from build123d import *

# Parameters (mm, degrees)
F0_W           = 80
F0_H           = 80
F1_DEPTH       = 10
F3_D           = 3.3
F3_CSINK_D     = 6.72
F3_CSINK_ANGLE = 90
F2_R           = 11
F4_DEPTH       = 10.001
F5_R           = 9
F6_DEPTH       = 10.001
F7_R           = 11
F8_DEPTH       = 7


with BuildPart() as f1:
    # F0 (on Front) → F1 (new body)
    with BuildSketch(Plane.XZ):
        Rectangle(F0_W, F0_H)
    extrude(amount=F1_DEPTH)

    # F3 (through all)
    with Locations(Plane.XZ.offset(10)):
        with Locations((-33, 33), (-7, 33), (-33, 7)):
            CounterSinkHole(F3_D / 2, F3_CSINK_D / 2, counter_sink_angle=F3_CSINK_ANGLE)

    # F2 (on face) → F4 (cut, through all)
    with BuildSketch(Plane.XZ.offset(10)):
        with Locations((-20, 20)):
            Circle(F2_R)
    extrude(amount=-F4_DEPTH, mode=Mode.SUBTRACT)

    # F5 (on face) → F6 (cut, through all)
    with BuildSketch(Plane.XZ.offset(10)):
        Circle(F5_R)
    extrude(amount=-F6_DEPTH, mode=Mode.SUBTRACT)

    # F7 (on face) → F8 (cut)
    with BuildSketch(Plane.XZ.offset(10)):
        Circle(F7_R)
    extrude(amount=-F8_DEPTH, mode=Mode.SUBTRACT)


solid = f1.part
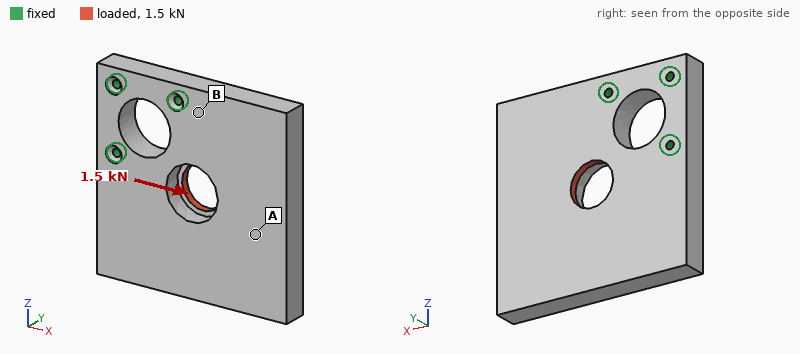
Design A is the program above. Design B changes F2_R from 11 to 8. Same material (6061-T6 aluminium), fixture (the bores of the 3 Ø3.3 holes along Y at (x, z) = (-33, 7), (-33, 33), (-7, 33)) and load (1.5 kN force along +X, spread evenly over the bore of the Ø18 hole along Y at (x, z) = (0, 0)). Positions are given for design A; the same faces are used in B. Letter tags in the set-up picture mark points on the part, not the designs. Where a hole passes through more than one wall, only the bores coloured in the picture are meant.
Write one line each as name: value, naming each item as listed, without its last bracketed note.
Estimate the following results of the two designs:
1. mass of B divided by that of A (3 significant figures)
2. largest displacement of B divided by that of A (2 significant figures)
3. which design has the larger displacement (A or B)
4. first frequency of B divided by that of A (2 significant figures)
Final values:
mass of B divided by that of A: 1.03
largest displacement of B divided by that of A: 0.89
which design has the larger displacement: A
first frequency of B divided by that of A: 1.0
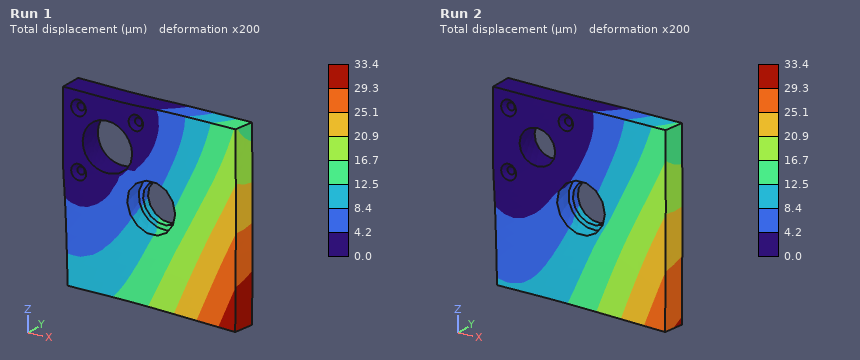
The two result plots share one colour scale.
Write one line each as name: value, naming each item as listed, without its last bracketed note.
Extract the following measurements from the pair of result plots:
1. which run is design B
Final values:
which run is design B: Run 2
